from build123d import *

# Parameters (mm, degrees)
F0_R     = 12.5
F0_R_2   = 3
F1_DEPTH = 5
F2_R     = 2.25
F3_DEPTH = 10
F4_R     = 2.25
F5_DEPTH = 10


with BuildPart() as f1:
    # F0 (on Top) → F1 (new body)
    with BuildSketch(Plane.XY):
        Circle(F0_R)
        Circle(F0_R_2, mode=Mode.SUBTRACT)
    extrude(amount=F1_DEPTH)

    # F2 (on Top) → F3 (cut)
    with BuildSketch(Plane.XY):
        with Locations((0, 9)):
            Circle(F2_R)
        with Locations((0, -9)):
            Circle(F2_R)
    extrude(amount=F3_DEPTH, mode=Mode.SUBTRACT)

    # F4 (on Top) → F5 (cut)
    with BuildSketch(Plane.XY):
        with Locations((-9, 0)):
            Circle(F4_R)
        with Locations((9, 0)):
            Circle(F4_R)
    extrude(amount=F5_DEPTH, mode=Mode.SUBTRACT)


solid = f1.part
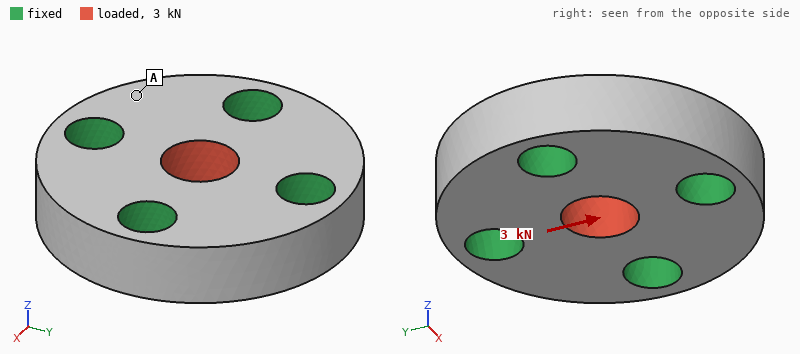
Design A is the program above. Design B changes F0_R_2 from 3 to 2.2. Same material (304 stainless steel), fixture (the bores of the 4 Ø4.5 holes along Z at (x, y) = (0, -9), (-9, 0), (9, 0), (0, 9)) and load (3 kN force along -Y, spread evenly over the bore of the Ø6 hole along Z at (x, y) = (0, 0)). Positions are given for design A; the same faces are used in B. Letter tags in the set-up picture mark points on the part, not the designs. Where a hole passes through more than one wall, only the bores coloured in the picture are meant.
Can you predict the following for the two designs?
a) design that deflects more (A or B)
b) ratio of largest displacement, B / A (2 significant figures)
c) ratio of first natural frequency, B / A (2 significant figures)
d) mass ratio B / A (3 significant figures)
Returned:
B
1.2
1.0
1.03
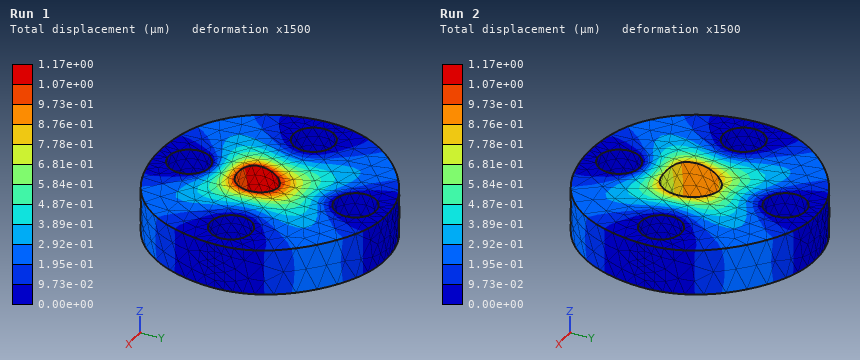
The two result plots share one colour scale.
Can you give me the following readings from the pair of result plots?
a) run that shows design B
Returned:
Run 1
